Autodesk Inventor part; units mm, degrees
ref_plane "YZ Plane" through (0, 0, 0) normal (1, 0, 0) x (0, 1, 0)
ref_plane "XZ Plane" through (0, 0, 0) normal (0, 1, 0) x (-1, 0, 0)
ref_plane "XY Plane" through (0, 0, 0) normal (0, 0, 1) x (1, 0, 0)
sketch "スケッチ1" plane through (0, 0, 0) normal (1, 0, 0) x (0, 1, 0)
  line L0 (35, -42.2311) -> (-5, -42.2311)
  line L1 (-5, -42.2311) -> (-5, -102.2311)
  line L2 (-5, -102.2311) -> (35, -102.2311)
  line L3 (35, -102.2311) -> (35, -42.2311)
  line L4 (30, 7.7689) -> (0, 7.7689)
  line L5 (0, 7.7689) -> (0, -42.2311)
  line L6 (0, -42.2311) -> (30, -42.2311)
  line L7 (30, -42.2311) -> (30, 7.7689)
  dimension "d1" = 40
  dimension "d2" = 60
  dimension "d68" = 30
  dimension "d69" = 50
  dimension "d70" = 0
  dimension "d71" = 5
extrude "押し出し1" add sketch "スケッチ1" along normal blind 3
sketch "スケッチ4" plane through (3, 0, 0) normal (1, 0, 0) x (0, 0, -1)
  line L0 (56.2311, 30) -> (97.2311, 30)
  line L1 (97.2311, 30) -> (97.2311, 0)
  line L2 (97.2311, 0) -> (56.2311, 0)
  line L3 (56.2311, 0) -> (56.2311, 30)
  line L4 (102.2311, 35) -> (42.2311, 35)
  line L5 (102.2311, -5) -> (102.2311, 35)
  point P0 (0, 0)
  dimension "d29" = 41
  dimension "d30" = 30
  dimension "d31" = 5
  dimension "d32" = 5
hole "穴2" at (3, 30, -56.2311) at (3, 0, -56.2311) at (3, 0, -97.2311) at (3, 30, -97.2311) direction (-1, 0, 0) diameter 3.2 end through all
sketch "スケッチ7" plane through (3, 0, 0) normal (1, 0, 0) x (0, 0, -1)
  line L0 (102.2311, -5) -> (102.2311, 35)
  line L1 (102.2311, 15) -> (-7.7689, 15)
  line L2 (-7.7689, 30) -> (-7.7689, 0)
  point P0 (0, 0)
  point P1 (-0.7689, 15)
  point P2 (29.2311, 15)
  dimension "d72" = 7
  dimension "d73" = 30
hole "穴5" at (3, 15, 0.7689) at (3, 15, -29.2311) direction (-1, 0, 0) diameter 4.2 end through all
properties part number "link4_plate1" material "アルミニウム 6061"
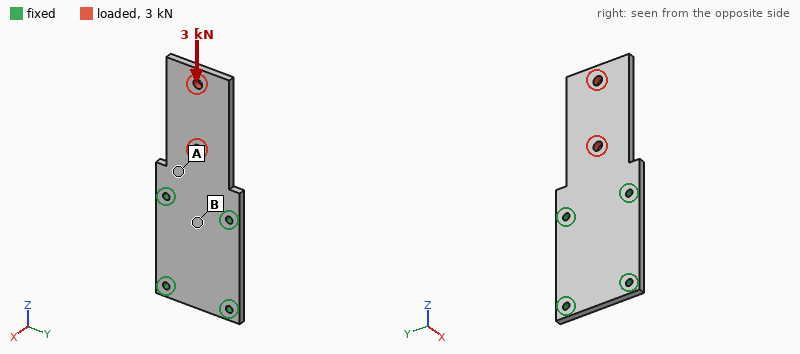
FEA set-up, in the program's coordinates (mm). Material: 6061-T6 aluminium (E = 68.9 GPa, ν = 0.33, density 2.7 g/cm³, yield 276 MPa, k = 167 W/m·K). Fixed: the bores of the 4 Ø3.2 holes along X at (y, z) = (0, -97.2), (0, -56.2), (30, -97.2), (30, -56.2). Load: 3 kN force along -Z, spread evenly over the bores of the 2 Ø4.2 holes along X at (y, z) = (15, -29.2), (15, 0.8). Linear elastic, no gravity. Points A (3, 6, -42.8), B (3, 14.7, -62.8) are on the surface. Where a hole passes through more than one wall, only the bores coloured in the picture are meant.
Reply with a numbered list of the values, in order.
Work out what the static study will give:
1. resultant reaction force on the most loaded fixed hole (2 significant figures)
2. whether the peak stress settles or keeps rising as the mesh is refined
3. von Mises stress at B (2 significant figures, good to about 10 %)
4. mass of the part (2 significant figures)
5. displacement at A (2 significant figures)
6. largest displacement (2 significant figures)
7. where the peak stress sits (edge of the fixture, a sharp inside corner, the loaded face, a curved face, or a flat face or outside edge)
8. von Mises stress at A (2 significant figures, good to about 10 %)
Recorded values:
1. 1.3 kN
2. keeps rising
3. 13 MPa
4. 31 g
5. 8.1 µm
6. 28 µm
7. edge of the fixture
8. 30 MPa
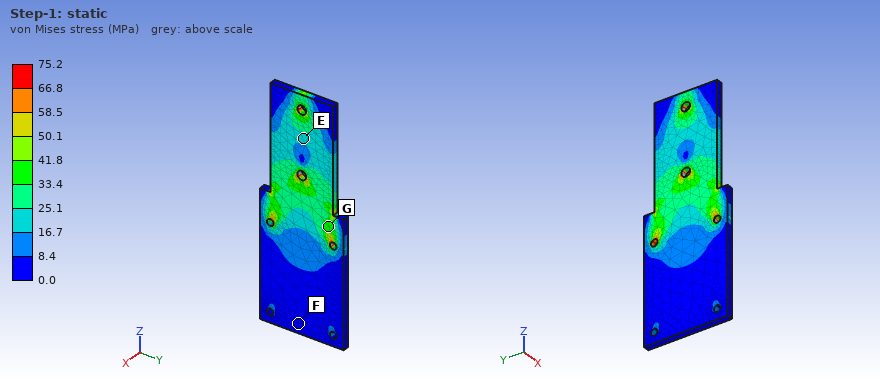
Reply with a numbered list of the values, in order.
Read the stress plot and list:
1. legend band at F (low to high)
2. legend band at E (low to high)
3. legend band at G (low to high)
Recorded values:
1. 0.0 to 8.4 MPa
2. 16.7 to 25.1 MPa
3. 33.4 to 41.8 MPa
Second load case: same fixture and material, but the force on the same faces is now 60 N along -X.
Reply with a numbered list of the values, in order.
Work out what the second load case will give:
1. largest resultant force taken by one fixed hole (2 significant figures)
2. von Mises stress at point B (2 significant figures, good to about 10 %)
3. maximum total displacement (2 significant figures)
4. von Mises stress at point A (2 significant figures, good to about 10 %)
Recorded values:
1. 37 N
2. 9.8 MPa
3. 0.57 mm
4. 35 MPa
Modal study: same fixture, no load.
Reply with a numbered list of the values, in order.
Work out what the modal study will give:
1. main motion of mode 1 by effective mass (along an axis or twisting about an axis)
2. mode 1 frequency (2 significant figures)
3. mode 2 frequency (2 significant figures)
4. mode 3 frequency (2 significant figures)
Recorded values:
1. along X
2. 630 Hz
3. 2800 Hz
4. 3700 Hz
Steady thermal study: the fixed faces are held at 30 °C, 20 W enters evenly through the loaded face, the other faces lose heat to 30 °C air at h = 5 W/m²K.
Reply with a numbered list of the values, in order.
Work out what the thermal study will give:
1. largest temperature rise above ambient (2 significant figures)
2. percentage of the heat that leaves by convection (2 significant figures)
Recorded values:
1. 59 K
2. 3.9 %
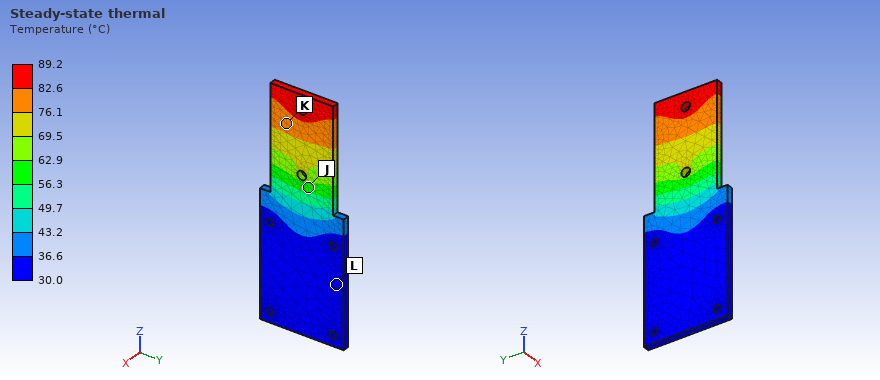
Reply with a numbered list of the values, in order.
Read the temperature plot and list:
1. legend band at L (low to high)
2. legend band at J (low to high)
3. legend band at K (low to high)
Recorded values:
1. 30.0 to 36.6 °C
2. 56.3 to 62.9 °C
3. 76.1 to 82.6 °C
